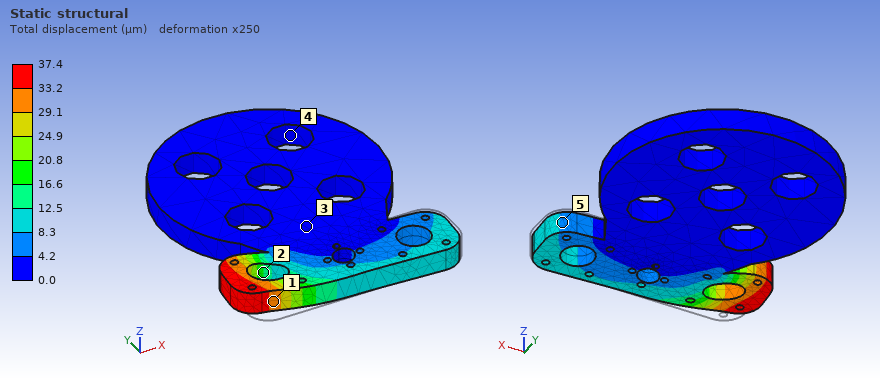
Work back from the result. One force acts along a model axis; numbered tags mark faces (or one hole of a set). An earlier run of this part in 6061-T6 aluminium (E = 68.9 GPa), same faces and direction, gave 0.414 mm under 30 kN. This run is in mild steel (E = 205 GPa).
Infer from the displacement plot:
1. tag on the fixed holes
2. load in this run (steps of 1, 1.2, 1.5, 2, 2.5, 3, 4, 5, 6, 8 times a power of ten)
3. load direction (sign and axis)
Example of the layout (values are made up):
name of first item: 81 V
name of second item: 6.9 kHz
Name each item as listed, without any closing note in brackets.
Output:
tag on the fixed holes: 4
load in this run: 8 kN
load direction: +Y
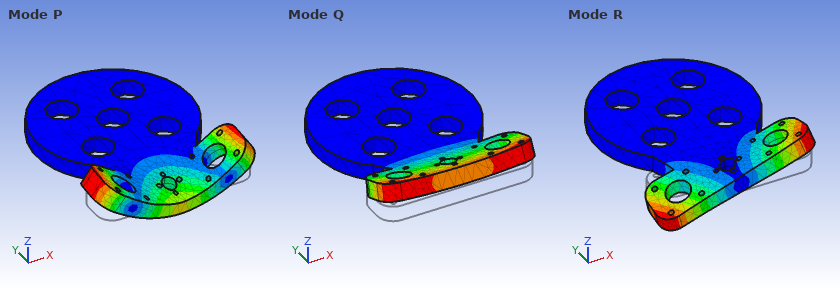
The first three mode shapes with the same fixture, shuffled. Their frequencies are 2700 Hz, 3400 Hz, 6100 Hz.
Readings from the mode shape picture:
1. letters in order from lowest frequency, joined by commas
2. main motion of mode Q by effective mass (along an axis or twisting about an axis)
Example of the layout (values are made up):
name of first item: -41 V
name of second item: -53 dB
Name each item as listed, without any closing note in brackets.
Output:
letters in order from lowest frequency, joined by commas: Q, R, P
main motion of mode Q by effective mass: along Z
